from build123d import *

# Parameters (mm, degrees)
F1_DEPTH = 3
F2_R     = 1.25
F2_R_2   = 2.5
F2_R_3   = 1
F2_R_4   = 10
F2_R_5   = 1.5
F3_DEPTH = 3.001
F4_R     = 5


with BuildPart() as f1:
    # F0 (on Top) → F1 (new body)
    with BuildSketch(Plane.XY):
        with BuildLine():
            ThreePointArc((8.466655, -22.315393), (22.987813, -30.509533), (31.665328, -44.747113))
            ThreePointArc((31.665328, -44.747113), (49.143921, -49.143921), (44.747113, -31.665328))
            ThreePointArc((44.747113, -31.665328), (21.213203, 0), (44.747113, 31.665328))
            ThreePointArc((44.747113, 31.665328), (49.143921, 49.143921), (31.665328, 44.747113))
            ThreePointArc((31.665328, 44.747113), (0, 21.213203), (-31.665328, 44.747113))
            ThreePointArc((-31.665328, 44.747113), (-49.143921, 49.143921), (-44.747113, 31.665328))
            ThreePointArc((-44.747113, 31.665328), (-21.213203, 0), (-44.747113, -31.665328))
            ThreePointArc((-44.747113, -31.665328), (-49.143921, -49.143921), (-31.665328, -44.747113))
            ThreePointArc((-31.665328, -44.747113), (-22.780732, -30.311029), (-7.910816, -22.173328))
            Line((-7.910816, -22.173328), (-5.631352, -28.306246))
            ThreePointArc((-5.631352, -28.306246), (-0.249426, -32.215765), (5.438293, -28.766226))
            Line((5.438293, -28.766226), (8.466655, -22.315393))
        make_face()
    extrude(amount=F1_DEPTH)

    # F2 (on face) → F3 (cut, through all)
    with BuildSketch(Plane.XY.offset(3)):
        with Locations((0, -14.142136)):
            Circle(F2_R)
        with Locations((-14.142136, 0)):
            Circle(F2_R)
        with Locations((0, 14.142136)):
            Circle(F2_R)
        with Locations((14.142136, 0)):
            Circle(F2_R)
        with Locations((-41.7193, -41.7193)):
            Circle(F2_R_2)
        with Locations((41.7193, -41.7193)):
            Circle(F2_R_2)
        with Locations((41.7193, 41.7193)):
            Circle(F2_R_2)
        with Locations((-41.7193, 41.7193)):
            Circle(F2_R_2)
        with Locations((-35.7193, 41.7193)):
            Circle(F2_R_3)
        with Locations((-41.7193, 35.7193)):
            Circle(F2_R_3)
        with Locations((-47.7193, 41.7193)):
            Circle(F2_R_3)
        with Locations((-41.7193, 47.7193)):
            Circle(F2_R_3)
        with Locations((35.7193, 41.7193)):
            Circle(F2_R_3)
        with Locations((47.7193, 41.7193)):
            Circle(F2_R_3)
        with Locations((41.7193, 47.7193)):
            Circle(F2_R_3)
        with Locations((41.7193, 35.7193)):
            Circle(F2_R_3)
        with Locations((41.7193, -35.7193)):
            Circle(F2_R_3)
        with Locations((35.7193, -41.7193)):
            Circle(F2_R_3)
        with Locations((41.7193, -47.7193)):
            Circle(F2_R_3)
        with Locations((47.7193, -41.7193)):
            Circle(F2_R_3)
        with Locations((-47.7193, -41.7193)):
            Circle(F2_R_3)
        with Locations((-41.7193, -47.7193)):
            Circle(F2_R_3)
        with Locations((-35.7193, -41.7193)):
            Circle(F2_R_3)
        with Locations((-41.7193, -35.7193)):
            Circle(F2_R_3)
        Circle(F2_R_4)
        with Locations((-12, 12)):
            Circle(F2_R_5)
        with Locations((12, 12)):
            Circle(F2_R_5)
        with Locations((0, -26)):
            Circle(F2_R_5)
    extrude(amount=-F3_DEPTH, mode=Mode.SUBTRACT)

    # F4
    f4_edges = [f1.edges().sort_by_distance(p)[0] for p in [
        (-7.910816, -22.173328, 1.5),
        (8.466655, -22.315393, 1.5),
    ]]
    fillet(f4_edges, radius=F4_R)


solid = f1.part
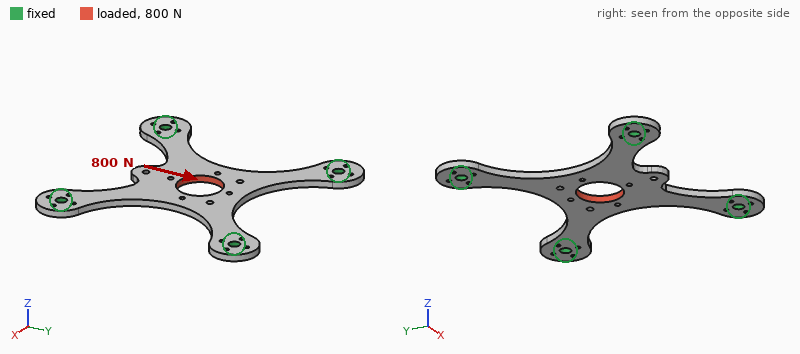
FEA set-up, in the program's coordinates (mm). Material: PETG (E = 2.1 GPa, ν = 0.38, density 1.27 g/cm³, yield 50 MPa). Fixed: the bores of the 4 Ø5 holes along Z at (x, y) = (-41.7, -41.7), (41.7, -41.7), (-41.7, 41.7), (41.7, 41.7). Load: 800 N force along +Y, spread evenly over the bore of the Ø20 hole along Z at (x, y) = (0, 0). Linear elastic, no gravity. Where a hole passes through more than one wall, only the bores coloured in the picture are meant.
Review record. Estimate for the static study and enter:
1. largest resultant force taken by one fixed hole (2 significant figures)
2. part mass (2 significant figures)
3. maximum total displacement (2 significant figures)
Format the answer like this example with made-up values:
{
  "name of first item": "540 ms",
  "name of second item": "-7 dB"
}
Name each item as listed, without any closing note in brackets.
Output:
{
  "largest resultant force taken by one fixed hole": "270 N",
  "part mass": "15 g",
  "maximum total displacement": "0.26 mm"
}
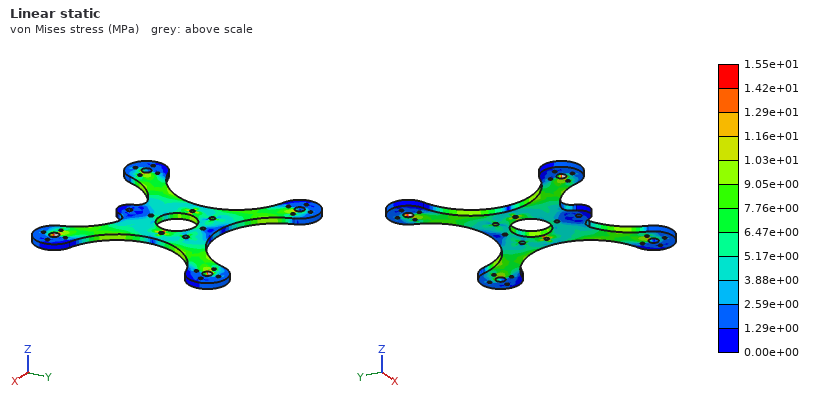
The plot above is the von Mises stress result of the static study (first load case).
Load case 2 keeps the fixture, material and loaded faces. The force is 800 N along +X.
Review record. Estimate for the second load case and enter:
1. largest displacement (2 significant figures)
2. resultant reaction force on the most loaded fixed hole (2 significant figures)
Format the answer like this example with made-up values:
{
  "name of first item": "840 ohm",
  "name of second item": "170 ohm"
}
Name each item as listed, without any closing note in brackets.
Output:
{
  "largest displacement": "0.25 mm",
  "resultant reaction force on the most loaded fixed hole": "270 N"
}
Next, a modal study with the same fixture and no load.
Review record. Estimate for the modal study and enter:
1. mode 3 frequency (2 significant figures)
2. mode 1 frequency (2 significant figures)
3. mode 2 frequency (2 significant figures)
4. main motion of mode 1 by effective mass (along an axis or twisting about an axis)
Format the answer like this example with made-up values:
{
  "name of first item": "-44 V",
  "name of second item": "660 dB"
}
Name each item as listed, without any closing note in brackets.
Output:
{
  "mode 3 frequency": "810 Hz",
  "mode 1 frequency": "350 Hz",
  "mode 2 frequency": "740 Hz",
  "main motion of mode 1 by effective mass": "along Z"
}
